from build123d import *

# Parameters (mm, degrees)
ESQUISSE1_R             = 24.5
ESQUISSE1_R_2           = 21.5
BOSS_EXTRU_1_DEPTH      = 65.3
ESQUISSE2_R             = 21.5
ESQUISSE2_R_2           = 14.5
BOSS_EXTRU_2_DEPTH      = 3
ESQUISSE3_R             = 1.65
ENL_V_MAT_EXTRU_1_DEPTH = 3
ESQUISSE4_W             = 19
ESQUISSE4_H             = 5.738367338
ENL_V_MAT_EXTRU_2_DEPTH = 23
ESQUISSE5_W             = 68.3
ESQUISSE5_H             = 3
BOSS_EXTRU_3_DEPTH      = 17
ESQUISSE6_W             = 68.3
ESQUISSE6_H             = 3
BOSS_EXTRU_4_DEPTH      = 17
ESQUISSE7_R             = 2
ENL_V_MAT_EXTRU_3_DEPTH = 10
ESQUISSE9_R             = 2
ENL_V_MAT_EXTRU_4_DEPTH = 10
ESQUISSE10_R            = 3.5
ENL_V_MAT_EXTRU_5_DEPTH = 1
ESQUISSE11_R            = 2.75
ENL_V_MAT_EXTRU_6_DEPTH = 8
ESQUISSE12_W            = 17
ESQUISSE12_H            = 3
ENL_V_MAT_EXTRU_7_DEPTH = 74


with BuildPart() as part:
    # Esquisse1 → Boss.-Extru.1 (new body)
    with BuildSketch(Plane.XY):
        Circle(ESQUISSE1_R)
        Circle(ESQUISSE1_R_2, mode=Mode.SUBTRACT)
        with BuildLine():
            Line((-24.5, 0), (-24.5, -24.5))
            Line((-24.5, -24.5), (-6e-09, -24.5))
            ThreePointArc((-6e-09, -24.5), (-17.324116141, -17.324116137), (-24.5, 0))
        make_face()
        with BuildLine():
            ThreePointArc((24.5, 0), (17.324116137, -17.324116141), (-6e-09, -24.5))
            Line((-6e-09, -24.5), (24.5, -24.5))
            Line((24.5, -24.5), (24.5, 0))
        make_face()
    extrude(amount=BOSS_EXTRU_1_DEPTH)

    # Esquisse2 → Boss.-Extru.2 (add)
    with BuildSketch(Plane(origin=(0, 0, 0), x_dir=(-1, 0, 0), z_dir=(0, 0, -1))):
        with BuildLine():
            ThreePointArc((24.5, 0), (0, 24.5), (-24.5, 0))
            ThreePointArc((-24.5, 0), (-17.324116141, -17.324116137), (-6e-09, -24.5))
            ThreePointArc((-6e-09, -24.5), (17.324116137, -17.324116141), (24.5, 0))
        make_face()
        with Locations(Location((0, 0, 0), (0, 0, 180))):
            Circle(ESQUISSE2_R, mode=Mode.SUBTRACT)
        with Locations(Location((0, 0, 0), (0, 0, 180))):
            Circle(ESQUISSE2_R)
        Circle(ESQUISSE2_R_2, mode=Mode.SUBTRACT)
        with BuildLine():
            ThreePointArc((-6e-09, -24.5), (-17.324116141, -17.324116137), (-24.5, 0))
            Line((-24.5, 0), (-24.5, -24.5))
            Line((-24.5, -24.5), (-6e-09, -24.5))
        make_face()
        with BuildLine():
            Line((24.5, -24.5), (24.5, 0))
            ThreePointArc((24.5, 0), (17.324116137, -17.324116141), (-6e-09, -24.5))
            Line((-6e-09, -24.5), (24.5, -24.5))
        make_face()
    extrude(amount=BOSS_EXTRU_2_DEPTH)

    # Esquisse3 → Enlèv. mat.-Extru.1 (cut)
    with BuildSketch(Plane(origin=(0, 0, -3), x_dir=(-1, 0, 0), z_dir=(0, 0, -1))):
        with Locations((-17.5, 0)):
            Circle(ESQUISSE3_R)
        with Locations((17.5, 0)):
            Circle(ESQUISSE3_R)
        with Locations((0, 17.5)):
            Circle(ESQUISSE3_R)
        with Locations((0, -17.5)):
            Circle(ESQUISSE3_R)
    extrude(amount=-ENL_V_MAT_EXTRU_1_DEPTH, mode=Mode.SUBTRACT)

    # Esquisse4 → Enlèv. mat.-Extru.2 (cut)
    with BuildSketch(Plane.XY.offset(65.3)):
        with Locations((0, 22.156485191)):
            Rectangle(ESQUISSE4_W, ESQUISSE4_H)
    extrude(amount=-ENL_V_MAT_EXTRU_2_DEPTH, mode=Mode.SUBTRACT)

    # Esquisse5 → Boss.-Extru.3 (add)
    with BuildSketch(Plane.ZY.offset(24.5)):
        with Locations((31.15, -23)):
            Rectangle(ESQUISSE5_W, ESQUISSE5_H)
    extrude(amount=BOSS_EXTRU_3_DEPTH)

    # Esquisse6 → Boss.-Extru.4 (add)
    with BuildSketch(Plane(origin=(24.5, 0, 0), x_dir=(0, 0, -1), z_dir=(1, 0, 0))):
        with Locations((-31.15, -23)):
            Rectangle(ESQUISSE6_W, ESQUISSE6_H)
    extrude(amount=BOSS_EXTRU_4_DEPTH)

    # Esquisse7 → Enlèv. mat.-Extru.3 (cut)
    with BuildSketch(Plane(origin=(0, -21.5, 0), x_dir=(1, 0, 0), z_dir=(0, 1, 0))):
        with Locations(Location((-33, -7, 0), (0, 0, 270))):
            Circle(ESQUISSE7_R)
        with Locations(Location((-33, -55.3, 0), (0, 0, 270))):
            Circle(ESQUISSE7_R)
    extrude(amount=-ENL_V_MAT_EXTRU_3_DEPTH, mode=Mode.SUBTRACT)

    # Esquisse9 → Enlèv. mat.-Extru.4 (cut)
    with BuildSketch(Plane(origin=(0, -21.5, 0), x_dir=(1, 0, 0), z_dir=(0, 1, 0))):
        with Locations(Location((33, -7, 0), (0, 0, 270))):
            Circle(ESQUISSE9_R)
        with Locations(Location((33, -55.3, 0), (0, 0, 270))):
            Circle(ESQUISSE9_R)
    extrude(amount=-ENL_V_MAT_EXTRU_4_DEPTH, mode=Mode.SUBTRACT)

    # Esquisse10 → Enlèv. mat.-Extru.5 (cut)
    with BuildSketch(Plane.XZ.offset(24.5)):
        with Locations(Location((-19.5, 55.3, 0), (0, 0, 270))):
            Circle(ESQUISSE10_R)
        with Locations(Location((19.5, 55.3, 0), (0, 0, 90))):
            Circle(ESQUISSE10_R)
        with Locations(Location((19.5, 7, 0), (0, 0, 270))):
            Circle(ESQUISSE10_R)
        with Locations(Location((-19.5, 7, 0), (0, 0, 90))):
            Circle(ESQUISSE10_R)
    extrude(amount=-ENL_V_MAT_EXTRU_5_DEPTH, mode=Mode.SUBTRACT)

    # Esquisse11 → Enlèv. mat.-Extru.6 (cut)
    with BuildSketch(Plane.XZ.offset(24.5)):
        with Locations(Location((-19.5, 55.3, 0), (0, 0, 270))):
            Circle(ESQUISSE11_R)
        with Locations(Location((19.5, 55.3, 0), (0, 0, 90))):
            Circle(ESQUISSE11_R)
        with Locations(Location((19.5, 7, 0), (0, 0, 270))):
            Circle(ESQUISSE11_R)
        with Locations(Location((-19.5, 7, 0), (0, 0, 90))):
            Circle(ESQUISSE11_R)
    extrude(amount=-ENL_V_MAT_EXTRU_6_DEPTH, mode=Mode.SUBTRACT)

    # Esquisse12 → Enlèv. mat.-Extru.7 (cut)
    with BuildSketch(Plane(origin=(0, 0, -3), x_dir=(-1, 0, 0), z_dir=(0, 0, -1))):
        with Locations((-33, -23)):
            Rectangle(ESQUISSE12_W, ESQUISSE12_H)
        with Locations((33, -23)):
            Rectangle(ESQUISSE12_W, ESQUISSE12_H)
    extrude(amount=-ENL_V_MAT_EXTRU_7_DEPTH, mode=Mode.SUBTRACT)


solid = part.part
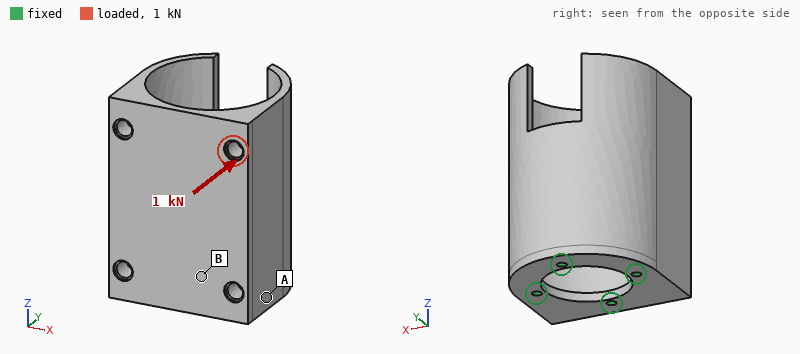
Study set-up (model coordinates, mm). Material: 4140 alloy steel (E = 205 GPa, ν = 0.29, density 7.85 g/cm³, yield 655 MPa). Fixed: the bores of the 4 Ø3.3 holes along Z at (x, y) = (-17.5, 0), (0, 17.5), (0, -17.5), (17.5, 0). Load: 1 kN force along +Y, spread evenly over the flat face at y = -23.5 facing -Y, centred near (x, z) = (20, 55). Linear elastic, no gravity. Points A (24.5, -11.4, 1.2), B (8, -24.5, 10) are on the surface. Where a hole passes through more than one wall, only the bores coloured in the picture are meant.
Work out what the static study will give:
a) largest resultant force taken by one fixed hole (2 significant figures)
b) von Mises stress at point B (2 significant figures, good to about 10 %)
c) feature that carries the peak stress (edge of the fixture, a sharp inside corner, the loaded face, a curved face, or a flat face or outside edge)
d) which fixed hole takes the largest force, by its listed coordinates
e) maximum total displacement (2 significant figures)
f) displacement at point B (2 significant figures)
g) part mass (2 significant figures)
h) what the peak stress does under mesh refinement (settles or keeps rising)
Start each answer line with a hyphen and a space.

- 1.5 kN
- 18 MPa
- edge of the fixture
- (0, -17.5)
- 45 µm
- 12 µm
- 370 g
- keeps rising
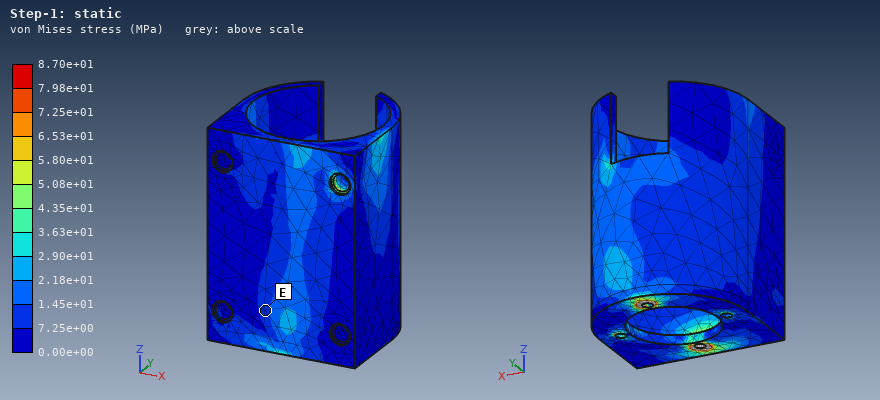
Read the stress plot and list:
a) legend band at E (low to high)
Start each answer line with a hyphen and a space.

- 7.25e+00 to 1.45e+01 MPa
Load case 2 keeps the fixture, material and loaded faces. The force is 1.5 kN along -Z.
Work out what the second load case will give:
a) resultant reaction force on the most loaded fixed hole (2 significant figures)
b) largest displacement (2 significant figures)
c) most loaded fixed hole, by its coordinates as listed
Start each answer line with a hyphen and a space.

- 1.3 kN
- 31 µm
- (0, -17.5)
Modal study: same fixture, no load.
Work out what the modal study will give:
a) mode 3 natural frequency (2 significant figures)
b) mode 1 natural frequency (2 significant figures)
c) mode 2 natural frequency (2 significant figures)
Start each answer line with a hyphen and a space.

- 4100 Hz
- 2300 Hz
- 2300 Hz
